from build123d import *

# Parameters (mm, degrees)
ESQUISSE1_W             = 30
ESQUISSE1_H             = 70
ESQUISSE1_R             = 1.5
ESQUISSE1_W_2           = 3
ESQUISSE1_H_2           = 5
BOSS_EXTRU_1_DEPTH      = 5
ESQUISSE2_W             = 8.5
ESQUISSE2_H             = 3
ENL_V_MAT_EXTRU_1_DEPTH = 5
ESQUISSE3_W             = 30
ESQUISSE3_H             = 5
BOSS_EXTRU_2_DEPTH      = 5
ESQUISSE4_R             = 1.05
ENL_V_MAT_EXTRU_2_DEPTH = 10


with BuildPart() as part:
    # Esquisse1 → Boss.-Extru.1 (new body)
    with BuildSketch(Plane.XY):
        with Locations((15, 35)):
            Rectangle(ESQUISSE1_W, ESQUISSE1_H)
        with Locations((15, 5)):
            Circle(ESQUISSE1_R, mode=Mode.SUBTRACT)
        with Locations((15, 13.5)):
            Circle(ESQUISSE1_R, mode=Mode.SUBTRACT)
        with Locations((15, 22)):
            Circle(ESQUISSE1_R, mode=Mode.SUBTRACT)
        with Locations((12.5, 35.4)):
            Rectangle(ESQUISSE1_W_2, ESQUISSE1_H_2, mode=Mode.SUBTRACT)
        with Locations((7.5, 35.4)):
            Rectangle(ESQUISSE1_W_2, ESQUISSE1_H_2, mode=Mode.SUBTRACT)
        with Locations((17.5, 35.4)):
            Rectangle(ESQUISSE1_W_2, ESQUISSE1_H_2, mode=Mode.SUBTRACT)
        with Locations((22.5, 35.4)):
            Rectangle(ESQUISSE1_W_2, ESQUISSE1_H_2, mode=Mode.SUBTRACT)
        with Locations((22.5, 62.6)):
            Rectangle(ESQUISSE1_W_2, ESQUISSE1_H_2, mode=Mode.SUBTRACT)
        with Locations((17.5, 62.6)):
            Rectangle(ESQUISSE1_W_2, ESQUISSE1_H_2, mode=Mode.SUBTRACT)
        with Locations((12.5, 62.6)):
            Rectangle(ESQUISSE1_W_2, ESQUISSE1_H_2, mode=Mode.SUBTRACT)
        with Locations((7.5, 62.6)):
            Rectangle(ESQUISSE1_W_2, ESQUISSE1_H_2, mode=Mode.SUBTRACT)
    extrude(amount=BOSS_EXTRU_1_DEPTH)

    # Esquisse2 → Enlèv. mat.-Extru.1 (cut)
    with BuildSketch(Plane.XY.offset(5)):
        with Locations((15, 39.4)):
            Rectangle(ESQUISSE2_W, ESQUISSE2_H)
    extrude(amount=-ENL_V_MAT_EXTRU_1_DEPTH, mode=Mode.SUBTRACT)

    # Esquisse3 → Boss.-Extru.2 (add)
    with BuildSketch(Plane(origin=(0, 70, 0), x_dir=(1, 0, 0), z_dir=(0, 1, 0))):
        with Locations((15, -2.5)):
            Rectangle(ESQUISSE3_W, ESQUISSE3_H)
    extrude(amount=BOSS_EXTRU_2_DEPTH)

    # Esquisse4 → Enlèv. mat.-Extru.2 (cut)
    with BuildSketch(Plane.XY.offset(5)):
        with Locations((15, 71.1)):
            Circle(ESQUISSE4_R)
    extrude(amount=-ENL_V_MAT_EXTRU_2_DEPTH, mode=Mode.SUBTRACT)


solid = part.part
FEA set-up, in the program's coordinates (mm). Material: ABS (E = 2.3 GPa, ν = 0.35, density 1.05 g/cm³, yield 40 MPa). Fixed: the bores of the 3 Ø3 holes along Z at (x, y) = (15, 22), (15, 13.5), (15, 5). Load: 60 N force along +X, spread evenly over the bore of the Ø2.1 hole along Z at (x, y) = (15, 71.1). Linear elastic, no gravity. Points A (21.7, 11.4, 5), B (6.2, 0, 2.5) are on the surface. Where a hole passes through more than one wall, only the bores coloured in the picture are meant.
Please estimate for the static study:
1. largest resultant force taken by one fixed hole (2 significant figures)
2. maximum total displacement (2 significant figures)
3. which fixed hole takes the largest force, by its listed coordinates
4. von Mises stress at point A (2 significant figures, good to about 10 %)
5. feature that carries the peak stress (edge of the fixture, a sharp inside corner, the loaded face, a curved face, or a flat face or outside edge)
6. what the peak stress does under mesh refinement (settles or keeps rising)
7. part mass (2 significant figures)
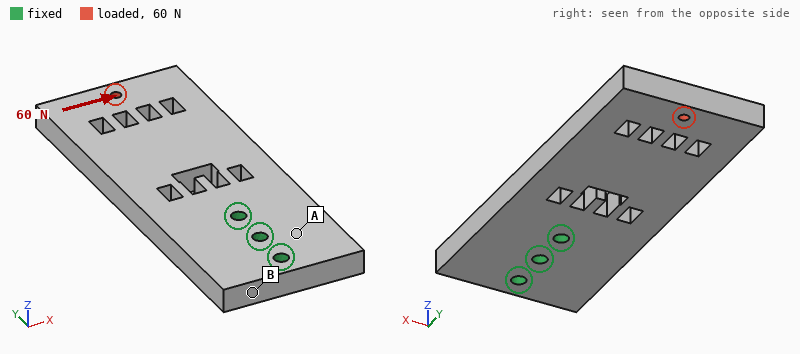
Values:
210 N
0.31 mm
(15, 22)
2.2 MPa
edge of the fixture
keeps rising
11 g
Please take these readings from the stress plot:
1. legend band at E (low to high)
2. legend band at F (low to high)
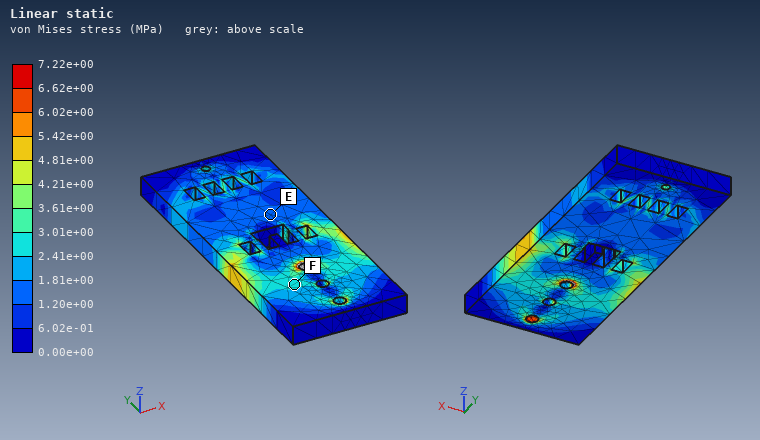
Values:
1.20e+00 to 1.81e+00 MPa
2.41e+00 to 3.01e+00 MPa
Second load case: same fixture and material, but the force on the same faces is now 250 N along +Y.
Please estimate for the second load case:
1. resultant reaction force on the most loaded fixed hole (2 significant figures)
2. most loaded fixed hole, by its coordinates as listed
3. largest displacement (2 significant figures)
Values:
140 N
(15, 22)
88 µm
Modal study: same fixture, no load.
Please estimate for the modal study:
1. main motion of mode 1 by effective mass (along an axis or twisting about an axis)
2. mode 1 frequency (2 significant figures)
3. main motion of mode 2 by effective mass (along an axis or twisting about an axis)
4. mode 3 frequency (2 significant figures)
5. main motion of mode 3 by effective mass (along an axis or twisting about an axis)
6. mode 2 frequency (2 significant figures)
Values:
along Z
370 Hz
twisting about Y
1300 Hz
along X
1200 Hz
